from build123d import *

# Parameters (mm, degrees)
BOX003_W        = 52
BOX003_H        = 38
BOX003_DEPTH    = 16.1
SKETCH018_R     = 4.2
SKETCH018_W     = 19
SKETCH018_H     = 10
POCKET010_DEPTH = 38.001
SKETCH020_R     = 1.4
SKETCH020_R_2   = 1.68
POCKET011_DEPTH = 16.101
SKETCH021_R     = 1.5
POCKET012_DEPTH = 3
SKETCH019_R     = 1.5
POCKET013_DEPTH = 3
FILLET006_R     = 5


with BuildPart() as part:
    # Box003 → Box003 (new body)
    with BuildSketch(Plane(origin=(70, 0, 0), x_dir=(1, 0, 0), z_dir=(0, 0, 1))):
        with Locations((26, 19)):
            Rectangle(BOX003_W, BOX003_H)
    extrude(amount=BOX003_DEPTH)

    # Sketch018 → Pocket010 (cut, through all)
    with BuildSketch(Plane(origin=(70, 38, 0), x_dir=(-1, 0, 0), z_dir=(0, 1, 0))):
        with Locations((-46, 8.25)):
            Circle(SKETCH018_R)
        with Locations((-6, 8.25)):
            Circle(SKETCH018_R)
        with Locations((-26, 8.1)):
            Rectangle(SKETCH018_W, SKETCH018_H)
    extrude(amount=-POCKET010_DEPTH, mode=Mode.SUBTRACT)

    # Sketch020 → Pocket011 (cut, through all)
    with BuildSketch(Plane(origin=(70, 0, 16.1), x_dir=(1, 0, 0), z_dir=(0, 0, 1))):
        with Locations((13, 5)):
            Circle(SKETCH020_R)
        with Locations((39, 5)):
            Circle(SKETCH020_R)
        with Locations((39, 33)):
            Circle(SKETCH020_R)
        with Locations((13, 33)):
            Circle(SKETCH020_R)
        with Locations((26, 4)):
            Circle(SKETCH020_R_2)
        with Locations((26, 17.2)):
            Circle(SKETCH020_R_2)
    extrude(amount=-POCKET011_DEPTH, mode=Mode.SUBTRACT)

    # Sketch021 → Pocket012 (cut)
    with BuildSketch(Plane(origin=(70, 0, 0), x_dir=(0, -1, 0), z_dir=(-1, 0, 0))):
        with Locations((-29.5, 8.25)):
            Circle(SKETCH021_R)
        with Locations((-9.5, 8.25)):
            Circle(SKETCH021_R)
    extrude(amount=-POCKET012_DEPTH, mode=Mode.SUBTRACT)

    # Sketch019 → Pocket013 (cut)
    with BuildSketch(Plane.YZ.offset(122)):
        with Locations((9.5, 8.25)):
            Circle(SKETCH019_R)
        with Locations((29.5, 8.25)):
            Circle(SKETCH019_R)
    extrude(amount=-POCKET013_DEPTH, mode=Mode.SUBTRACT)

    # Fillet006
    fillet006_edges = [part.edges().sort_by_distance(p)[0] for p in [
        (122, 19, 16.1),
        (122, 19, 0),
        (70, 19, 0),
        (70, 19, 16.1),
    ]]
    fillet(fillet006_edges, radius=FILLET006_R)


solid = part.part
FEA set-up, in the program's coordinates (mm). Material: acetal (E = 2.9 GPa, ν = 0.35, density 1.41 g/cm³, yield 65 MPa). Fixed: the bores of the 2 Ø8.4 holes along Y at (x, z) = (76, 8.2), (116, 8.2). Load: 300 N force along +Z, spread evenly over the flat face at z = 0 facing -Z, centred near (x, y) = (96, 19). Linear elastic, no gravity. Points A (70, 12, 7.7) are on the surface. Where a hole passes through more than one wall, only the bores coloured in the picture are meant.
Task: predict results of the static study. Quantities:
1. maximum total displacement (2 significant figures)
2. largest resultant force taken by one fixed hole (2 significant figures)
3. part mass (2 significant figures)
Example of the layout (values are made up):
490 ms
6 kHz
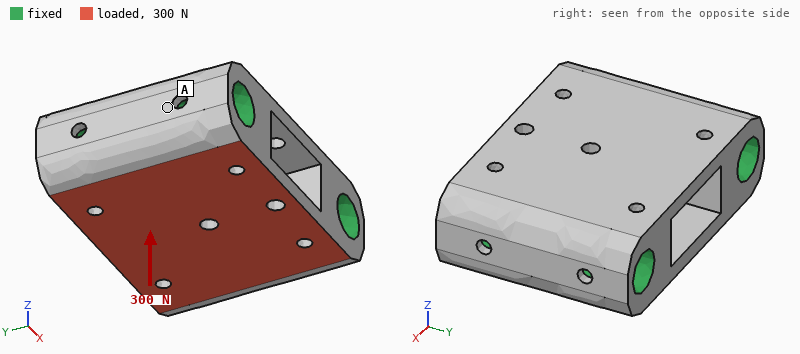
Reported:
26 µm
150 N
27 g
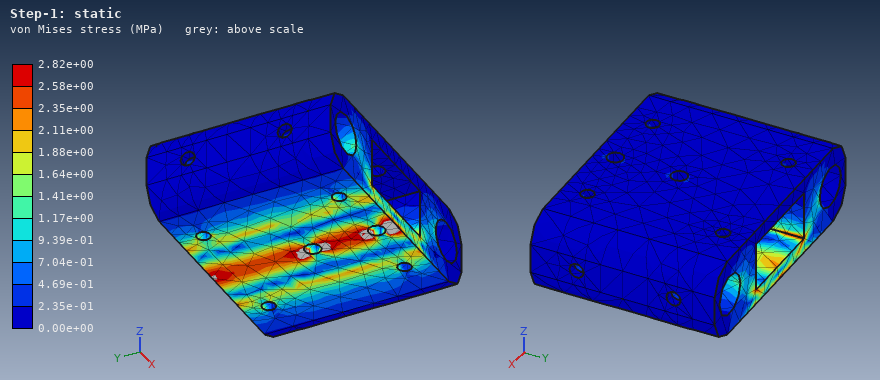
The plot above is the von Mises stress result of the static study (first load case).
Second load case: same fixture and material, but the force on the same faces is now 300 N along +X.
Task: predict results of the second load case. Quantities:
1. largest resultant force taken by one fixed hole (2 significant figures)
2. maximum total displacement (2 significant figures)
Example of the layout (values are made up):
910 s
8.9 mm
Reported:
150 N
4.0 µm
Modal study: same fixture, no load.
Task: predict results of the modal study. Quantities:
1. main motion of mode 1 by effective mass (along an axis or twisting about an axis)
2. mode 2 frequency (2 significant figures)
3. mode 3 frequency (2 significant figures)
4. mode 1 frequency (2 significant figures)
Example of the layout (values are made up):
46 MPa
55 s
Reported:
along Z
8200 Hz
8400 Hz
7800 Hz
